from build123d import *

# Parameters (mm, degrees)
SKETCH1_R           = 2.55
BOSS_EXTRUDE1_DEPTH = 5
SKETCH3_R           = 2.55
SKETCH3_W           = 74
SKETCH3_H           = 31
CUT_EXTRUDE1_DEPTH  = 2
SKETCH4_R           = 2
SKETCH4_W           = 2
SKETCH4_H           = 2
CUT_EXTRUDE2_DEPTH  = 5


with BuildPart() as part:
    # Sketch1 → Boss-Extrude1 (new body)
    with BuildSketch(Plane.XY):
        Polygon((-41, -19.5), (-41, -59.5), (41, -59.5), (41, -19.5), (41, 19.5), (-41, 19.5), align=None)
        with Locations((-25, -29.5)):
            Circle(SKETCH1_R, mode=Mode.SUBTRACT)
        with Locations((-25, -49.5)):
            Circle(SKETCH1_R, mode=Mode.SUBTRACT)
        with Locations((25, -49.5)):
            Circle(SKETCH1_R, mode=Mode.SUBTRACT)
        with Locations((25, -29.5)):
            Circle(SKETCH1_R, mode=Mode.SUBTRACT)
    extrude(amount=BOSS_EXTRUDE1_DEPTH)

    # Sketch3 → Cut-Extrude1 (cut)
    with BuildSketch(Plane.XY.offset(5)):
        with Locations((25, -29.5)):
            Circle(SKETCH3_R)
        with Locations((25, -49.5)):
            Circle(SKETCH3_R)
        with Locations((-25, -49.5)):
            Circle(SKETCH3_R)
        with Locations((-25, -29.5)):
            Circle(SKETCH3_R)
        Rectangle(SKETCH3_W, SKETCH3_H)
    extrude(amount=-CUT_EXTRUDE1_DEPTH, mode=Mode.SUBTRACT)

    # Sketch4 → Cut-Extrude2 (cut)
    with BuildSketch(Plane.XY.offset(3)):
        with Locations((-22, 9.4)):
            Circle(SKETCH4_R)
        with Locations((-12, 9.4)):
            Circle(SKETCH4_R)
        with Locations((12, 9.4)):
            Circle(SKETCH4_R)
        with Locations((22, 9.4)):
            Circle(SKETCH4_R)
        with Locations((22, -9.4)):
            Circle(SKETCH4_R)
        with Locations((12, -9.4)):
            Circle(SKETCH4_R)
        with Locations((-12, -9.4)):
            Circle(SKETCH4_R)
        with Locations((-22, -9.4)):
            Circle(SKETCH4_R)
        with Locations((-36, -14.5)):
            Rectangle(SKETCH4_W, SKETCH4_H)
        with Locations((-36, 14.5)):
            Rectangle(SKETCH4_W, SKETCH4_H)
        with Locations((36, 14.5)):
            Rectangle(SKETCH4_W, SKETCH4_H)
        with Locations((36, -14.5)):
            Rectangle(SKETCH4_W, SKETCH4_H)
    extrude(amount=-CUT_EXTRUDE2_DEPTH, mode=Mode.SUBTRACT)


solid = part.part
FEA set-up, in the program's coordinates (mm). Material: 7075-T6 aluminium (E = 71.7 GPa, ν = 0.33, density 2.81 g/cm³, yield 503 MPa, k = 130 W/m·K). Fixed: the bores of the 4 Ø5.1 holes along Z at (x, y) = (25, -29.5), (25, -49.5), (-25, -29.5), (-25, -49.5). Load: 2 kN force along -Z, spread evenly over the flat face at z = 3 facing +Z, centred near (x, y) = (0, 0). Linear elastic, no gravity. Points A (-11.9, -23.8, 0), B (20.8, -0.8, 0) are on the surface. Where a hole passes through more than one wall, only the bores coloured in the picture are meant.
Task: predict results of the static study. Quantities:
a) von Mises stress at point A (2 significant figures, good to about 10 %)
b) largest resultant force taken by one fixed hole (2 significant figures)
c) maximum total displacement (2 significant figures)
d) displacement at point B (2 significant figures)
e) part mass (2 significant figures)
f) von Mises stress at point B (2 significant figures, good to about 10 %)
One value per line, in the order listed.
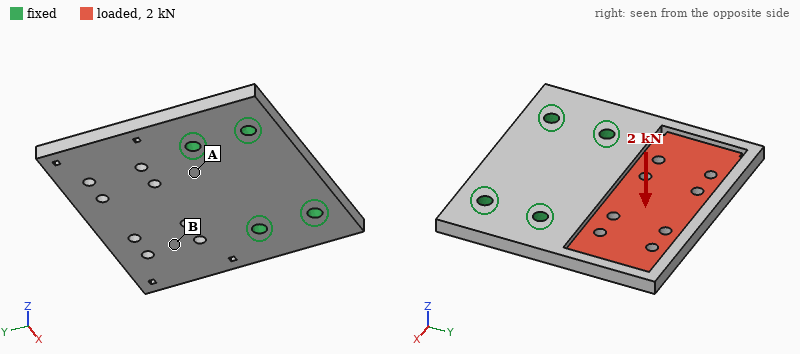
100 MPa
1.6 kN
1.1 mm
0.45 mm
76 g
40 MPa
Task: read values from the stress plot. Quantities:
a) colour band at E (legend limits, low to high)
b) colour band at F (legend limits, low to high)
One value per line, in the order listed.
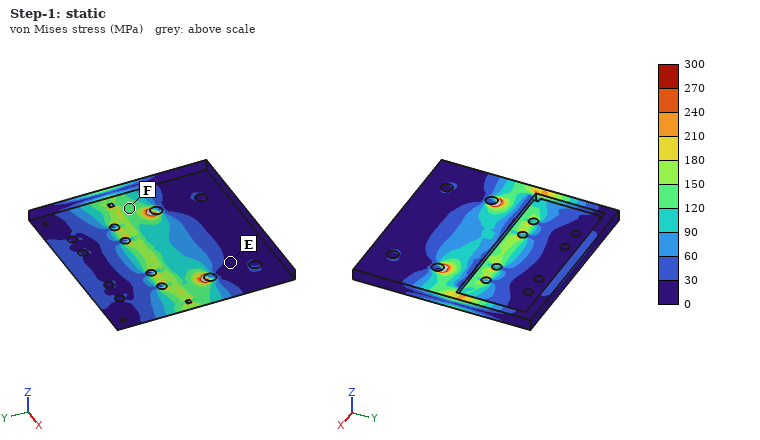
0 to 30 MPa
120 to 150 MPa
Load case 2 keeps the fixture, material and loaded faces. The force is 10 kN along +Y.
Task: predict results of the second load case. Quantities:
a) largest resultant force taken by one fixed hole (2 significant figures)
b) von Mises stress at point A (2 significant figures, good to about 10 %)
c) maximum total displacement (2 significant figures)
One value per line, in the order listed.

3.6 kN
18 MPa
0.43 mm
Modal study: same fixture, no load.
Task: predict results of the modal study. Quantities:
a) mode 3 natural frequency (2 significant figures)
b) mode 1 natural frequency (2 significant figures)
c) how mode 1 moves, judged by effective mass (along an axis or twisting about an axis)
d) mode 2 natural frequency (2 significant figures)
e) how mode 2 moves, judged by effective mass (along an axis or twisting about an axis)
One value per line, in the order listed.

4400 Hz
1500 Hz
along Z
2200 Hz
twisting about Y
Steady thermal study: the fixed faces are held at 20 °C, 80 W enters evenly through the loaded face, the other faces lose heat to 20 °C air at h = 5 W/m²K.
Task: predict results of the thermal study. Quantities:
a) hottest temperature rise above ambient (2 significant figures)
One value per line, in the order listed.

71 K
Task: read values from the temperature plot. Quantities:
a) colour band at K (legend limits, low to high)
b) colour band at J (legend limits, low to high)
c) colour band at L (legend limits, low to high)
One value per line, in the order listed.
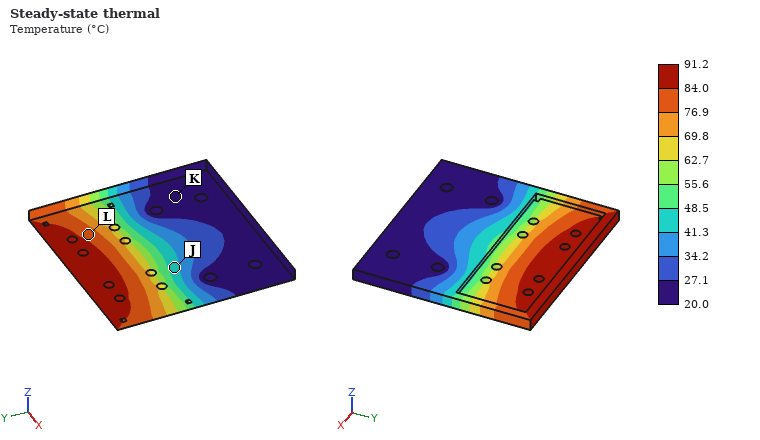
20.0 to 27.1 °C
41.3 to 48.5 °C
76.9 to 84.0 °C
